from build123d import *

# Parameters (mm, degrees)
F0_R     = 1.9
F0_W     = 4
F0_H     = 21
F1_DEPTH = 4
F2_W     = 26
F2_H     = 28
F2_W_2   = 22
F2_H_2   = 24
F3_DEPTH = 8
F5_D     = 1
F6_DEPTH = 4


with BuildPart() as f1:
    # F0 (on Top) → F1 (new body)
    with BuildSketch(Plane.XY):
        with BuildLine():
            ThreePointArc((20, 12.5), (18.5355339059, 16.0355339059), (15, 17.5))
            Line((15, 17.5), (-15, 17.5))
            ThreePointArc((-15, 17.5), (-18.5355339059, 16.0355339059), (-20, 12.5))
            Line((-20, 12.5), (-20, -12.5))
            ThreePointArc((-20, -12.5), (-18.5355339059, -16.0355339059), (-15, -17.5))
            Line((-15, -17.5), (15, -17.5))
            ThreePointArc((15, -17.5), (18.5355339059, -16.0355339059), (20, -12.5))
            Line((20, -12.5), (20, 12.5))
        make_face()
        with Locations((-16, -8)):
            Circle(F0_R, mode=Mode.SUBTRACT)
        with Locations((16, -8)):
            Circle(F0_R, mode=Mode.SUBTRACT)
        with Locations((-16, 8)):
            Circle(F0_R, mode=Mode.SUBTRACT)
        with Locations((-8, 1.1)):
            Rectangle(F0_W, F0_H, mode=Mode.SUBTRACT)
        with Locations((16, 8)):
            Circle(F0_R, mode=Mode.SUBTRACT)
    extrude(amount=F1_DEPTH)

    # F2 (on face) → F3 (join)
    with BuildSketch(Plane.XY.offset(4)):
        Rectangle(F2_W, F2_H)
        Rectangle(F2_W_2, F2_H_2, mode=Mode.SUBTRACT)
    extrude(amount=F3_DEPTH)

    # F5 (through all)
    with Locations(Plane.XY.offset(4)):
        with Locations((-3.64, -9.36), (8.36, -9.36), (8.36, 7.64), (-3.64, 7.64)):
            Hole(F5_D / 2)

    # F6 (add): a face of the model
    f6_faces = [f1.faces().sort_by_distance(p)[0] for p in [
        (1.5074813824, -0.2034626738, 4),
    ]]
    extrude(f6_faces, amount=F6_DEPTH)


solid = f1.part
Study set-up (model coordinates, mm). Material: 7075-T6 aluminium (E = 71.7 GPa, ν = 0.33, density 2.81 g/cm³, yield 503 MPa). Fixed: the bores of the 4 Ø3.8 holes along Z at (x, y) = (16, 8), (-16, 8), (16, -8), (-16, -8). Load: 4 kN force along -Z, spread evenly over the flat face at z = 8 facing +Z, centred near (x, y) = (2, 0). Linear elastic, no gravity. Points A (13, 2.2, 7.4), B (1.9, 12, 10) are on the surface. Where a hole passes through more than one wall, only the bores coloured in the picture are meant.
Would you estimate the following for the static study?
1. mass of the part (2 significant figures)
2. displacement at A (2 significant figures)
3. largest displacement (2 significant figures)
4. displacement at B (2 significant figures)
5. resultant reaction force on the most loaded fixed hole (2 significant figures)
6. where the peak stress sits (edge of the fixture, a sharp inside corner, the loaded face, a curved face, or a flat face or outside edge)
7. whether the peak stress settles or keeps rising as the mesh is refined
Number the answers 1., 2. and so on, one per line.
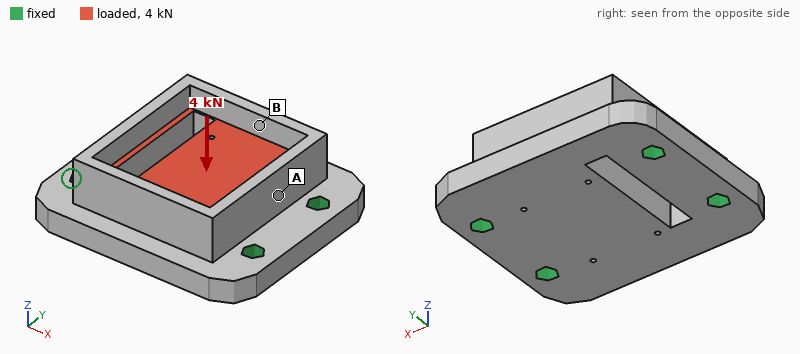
1. 23 g
2. 9.1 µm
3. 32 µm
4. 18 µm
5. 1.2 kN
6. edge of the fixture
7. keeps rising
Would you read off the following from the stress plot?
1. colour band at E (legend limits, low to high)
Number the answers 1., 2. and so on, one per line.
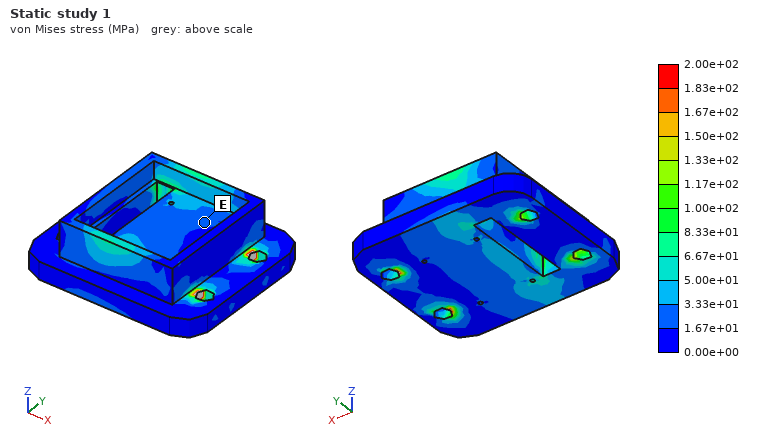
1. 1.67e+01 to 3.33e+01 MPa
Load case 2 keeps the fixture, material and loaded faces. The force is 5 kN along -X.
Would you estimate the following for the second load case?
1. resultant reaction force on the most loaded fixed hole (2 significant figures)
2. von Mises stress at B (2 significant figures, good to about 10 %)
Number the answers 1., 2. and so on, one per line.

1. 1.9 kN
2. 20 MPa
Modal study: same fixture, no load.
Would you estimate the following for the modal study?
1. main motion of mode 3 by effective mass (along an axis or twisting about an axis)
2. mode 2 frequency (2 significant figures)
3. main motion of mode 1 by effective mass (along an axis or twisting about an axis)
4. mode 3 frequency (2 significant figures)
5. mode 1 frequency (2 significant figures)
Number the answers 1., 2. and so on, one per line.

1. along Y
2. 20 kHz
3. along Z
4. 28 kHz
5. 19 kHz
